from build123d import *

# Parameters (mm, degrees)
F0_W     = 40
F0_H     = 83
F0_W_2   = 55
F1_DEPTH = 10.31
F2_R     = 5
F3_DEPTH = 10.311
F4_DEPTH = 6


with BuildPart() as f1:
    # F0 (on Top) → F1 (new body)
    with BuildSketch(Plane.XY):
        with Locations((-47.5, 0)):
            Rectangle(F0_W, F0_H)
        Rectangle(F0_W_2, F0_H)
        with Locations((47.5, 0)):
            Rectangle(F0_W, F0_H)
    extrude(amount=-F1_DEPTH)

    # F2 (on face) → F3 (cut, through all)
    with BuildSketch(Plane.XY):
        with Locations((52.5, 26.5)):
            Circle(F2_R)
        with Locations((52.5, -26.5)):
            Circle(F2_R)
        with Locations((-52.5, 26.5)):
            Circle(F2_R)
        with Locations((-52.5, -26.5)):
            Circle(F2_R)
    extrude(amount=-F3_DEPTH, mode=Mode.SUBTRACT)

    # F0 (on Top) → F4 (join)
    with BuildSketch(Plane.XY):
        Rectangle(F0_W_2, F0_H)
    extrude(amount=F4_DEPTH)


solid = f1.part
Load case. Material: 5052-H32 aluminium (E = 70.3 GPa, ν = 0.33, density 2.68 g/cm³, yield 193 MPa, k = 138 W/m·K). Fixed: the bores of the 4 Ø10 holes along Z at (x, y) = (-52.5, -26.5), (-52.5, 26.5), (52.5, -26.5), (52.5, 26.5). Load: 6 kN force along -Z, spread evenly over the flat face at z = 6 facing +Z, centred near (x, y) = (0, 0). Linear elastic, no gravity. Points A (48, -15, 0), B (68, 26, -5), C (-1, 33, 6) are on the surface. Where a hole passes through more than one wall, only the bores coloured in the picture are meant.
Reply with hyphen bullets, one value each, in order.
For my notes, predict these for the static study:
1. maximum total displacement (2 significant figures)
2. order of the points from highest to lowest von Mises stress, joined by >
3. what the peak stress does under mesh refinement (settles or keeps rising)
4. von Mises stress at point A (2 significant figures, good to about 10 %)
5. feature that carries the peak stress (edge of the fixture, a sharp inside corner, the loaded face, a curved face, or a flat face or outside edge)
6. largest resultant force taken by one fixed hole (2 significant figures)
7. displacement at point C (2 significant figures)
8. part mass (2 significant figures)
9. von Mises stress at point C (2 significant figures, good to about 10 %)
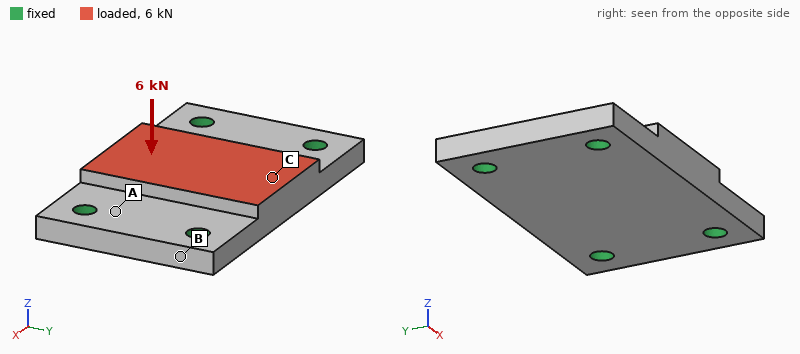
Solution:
- 32 µm
- C > A > B
- keeps rising
- 12 MPa
- edge of the fixture
- 1.8 kN
- 30 µm
- 370 g
- 17 MPa
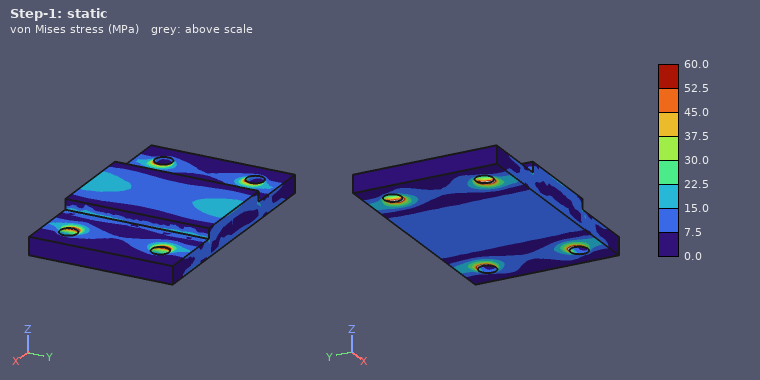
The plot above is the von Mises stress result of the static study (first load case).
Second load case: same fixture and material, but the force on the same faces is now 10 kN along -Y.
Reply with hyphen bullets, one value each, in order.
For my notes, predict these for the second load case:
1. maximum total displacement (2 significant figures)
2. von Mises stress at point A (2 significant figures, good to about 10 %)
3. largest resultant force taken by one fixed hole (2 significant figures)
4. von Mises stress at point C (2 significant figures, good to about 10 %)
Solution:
- 34 µm
- 16 MPa
- 3.3 kN
- 8.5 MPa
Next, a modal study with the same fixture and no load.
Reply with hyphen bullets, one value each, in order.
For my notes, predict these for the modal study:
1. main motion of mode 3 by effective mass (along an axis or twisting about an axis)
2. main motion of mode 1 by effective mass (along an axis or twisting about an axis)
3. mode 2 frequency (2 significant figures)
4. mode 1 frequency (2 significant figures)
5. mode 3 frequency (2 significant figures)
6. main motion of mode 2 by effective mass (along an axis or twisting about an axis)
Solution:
- along Y
- along Z
- 6200 Hz
- 5100 Hz
- 11 kHz
- twisting about X
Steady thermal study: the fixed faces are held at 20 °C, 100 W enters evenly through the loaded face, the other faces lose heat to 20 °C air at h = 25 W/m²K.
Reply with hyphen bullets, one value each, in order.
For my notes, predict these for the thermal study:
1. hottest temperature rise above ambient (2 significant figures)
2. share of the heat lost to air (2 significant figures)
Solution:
- 16 K
- 4.1 %
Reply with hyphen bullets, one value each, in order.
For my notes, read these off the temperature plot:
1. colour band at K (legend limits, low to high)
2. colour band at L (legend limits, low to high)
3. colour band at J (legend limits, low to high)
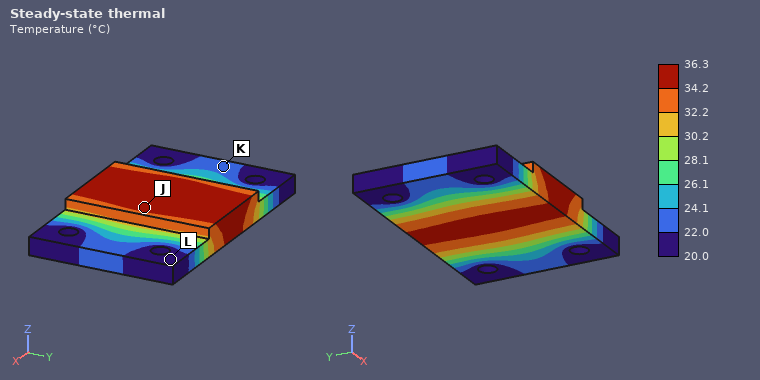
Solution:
- 22.0 to 24.1 °C
- 20.0 to 22.0 °C
- 34.2 to 36.3 °C
